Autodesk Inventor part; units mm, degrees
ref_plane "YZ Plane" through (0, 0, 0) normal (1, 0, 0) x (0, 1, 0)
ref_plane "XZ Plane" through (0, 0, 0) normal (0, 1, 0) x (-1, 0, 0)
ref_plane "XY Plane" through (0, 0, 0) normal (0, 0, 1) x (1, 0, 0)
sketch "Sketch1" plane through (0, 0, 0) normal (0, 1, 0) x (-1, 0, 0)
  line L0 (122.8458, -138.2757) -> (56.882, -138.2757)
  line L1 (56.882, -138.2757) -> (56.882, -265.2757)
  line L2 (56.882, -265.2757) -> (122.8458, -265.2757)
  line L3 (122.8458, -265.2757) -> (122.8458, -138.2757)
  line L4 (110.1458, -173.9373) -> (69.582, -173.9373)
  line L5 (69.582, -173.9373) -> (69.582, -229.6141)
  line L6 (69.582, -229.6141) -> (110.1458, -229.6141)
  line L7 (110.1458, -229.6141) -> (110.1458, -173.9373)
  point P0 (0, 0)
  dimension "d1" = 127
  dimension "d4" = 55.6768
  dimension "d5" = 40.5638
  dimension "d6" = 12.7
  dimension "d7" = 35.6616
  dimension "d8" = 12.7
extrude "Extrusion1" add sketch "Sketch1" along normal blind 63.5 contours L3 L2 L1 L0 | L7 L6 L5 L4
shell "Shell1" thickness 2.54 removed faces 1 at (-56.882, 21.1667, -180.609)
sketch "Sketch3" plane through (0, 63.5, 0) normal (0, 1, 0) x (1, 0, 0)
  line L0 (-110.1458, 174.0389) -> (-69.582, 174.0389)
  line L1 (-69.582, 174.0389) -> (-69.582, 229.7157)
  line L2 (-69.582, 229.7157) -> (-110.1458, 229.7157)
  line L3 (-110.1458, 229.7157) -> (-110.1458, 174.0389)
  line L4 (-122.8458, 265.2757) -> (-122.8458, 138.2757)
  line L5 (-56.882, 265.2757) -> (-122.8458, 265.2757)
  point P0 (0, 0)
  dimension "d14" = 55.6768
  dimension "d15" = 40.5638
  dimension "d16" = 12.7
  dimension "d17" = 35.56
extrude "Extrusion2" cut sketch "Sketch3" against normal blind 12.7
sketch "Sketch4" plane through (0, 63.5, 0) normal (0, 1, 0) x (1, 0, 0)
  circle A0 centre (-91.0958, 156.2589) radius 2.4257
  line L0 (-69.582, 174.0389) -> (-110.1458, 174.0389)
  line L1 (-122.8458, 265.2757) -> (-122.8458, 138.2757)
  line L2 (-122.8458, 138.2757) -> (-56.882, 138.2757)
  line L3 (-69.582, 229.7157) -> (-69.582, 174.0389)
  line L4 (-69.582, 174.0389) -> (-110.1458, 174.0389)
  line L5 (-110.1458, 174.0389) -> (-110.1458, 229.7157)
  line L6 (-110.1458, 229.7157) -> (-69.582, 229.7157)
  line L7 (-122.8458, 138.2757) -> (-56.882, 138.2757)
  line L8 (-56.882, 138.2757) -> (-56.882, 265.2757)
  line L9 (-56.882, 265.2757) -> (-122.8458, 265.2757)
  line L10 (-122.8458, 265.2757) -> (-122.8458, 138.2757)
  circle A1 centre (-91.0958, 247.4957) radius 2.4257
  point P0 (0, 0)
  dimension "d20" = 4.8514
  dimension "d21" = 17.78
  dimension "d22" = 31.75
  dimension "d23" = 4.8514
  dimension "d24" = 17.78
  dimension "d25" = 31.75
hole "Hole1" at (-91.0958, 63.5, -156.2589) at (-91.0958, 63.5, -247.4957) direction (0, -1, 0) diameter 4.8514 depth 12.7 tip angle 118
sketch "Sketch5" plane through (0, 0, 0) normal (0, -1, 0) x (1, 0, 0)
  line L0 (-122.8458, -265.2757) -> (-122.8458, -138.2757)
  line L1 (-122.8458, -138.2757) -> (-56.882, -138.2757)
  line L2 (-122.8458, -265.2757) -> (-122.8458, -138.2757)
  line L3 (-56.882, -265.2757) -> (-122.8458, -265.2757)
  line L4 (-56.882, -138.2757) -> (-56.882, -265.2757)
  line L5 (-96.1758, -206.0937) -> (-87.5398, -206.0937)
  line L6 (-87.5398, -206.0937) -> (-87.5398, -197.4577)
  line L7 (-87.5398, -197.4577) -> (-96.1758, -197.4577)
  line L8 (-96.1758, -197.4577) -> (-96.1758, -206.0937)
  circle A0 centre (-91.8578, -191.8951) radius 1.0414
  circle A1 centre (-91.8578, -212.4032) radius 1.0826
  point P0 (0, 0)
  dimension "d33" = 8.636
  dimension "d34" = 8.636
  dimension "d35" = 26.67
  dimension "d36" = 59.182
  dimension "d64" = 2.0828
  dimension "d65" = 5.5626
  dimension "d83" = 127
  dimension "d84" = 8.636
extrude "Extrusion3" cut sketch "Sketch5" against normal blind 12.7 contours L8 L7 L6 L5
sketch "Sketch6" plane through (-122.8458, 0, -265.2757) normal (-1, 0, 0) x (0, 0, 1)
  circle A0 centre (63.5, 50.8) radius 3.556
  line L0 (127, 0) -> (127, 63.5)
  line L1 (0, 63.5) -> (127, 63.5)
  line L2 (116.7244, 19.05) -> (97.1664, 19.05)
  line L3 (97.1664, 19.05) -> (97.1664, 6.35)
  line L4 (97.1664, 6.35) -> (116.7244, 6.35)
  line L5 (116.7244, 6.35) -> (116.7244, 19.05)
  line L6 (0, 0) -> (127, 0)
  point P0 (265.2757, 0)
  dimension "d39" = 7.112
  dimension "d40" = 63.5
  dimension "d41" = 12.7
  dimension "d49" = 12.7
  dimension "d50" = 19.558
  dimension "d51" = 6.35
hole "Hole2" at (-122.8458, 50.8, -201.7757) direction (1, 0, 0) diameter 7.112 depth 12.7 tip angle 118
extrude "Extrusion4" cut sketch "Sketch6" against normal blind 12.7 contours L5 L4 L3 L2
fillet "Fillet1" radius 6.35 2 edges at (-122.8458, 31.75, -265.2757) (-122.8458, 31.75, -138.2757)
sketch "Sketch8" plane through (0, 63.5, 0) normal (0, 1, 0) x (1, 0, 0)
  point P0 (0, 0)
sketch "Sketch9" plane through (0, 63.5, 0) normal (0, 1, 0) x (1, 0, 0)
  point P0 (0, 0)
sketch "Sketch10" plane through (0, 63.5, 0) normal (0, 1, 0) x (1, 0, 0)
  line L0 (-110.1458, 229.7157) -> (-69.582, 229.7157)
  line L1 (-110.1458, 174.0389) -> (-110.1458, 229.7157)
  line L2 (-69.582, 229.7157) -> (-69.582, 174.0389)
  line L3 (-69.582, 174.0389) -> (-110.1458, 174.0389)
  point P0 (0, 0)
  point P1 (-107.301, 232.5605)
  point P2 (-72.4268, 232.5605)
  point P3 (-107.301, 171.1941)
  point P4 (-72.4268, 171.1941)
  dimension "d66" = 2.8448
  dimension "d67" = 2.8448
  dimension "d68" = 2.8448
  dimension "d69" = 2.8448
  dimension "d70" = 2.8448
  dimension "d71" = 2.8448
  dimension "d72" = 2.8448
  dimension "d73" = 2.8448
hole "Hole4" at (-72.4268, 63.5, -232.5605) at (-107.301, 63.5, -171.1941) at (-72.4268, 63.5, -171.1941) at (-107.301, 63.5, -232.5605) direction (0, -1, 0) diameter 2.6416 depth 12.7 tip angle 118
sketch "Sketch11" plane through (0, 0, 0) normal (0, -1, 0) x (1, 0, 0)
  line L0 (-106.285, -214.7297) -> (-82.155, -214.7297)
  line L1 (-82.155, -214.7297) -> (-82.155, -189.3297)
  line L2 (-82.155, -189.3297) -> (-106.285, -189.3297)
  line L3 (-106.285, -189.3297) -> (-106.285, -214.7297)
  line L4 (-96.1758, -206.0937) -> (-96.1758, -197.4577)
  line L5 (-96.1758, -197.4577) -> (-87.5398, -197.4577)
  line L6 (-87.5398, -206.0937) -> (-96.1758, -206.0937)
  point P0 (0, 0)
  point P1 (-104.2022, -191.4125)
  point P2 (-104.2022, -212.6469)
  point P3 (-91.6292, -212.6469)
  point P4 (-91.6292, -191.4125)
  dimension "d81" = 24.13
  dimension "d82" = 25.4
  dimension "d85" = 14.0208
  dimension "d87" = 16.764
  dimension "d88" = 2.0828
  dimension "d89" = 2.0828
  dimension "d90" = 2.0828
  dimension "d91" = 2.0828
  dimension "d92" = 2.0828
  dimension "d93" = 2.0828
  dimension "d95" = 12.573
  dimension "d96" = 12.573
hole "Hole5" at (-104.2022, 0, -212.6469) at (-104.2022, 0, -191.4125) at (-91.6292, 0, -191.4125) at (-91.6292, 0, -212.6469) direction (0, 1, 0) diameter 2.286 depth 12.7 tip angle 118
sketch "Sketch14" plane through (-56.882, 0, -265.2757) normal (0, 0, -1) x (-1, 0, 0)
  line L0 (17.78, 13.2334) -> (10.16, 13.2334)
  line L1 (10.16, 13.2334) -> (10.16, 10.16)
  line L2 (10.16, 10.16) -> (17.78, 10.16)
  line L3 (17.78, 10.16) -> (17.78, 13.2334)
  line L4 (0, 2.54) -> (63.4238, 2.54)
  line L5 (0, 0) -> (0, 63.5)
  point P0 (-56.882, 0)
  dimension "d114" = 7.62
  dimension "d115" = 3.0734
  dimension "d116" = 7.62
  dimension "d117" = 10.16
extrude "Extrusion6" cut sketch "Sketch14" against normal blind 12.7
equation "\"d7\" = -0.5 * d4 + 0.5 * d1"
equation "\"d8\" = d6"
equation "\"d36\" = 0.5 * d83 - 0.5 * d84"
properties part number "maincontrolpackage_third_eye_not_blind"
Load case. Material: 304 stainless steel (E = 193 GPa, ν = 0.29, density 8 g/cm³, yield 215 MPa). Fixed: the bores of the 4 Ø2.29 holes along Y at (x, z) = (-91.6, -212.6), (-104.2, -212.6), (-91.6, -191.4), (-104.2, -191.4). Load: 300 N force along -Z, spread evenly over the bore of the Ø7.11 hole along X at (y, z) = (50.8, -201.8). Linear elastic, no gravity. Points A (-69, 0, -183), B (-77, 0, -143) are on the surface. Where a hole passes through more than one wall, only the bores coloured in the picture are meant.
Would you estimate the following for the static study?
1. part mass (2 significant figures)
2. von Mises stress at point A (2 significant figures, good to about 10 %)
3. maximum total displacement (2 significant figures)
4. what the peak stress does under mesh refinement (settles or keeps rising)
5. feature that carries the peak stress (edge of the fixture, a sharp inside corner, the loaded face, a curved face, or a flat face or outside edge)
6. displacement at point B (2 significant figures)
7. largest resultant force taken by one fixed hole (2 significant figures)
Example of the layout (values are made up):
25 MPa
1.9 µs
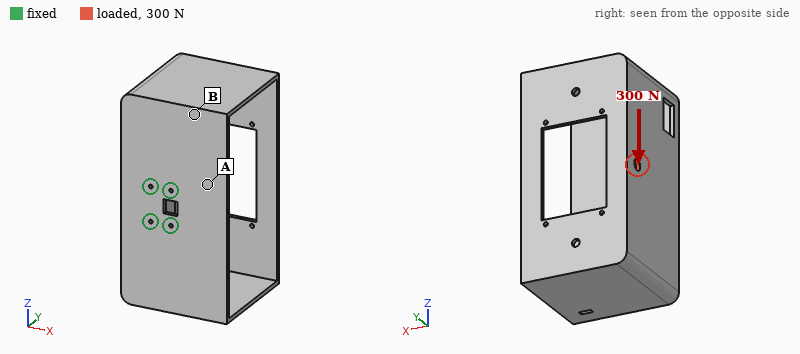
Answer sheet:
580 g
21 MPa
0.27 mm
keeps rising
edge of the fixture
0.13 mm
490 N
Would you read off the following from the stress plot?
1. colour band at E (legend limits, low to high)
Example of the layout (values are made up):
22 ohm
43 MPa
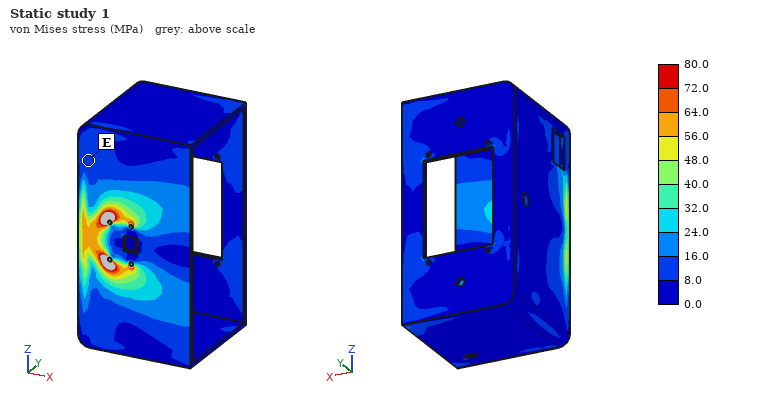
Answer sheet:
8.0 to 16.0 MPa
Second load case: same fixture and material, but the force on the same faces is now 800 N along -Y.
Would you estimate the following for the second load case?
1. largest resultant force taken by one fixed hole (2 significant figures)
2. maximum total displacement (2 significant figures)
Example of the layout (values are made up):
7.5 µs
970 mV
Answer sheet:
670 N
0.24 mm
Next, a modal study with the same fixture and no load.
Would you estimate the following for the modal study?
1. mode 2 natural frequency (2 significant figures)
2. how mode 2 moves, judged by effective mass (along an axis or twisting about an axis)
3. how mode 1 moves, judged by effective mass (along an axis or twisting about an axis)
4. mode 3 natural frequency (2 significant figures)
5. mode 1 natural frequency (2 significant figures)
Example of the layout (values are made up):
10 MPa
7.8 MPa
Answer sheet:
260 Hz
along Z
along X
440 Hz
230 Hz
